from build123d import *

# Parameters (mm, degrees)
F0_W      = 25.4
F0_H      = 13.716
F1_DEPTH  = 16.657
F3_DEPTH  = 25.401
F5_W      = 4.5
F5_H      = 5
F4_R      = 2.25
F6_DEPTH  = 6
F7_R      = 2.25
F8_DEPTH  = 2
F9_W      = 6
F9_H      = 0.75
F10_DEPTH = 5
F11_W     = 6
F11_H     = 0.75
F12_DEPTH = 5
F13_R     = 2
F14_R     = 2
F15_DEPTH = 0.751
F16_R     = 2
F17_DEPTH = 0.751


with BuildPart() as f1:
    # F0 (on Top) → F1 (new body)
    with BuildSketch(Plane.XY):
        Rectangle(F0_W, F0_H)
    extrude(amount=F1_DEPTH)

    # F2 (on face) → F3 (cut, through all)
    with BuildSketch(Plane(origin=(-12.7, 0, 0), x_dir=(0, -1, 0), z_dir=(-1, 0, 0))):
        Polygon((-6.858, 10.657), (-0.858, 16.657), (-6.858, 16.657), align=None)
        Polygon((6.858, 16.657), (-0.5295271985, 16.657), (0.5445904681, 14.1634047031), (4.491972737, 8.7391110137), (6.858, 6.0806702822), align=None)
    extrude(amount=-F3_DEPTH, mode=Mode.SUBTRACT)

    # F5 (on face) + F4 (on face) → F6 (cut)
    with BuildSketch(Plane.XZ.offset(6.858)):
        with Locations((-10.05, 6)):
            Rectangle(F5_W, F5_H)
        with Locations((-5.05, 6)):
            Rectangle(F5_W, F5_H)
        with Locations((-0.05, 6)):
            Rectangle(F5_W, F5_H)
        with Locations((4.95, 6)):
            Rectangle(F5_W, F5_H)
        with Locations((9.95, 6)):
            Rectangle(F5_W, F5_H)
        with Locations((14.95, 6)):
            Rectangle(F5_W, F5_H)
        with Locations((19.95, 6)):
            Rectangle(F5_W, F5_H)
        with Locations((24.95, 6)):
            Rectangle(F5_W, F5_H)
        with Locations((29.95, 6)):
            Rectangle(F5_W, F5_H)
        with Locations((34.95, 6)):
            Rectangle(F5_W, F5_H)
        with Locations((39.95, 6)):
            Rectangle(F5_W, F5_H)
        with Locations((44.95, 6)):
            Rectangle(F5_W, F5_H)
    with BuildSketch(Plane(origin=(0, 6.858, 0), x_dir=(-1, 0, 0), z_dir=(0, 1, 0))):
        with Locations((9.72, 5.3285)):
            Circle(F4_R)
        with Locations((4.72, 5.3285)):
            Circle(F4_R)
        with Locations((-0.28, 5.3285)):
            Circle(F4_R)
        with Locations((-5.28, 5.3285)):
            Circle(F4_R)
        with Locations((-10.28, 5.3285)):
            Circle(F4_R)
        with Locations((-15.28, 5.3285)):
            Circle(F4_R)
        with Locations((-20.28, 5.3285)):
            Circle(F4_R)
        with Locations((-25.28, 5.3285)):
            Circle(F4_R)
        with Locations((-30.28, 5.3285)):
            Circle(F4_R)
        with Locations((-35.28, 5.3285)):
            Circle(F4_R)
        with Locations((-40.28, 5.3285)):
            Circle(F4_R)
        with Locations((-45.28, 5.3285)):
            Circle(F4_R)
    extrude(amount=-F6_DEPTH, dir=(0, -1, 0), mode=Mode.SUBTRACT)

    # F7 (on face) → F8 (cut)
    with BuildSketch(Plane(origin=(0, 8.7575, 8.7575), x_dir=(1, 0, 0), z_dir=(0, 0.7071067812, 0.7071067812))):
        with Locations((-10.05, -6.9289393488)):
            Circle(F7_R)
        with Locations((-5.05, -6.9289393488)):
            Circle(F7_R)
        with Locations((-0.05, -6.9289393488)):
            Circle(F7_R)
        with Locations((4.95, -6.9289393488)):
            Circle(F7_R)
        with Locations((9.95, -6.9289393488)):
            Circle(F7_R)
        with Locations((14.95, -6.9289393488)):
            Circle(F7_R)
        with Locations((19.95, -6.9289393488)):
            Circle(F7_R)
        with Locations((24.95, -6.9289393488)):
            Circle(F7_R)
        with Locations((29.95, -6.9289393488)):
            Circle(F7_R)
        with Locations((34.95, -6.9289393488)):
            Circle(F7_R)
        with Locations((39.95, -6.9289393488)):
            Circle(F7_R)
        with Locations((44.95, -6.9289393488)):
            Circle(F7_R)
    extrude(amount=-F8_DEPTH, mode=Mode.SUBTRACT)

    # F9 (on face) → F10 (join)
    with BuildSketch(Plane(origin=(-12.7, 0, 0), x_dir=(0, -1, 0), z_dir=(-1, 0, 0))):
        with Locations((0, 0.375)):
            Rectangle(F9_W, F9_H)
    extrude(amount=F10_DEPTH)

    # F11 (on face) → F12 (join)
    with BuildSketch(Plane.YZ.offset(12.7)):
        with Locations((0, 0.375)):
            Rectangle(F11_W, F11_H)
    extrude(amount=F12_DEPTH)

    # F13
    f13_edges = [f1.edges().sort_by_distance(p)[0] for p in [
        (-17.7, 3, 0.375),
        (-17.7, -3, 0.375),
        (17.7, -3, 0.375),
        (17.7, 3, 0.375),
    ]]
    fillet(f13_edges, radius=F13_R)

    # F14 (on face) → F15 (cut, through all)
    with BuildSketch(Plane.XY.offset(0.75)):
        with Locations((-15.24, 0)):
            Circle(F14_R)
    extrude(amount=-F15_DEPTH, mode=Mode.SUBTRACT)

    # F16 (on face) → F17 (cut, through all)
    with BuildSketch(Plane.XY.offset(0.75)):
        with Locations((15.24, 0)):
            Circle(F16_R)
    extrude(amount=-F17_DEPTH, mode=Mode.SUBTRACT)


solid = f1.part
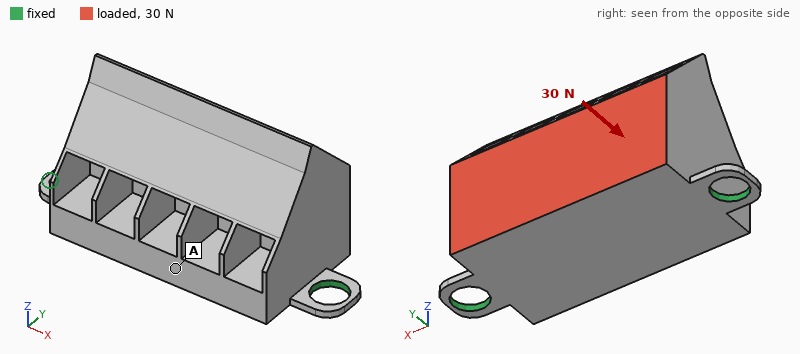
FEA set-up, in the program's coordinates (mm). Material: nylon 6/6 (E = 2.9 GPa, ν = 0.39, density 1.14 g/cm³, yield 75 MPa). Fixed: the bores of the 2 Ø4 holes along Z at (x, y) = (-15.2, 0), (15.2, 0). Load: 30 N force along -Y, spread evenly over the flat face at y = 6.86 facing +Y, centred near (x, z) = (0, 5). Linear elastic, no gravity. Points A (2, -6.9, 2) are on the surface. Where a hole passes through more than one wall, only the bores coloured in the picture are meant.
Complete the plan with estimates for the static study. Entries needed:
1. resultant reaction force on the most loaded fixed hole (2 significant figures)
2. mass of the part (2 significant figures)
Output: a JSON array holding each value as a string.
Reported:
["15 N", "4.0 g"]
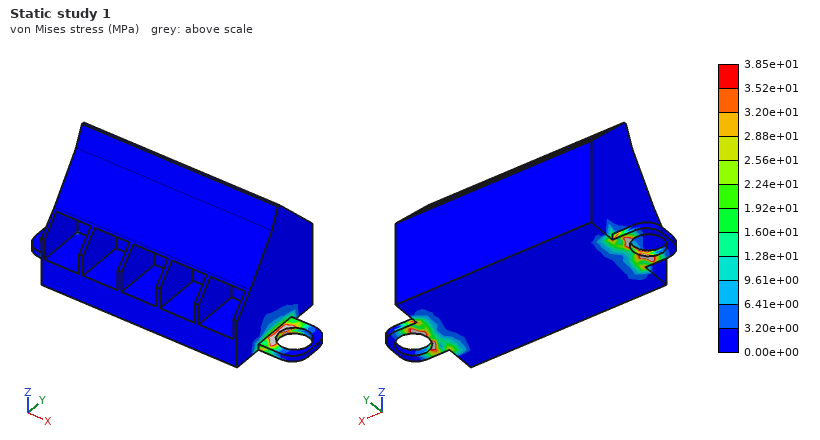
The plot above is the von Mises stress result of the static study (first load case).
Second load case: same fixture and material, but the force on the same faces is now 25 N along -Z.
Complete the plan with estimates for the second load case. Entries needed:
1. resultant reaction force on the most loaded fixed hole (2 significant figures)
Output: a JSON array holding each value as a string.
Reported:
["15 N"]
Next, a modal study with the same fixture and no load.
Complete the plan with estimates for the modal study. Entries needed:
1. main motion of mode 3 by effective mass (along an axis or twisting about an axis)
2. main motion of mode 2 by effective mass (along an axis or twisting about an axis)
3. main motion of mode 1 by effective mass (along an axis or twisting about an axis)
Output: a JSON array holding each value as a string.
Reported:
["along X", "along Z", "along Y"]
